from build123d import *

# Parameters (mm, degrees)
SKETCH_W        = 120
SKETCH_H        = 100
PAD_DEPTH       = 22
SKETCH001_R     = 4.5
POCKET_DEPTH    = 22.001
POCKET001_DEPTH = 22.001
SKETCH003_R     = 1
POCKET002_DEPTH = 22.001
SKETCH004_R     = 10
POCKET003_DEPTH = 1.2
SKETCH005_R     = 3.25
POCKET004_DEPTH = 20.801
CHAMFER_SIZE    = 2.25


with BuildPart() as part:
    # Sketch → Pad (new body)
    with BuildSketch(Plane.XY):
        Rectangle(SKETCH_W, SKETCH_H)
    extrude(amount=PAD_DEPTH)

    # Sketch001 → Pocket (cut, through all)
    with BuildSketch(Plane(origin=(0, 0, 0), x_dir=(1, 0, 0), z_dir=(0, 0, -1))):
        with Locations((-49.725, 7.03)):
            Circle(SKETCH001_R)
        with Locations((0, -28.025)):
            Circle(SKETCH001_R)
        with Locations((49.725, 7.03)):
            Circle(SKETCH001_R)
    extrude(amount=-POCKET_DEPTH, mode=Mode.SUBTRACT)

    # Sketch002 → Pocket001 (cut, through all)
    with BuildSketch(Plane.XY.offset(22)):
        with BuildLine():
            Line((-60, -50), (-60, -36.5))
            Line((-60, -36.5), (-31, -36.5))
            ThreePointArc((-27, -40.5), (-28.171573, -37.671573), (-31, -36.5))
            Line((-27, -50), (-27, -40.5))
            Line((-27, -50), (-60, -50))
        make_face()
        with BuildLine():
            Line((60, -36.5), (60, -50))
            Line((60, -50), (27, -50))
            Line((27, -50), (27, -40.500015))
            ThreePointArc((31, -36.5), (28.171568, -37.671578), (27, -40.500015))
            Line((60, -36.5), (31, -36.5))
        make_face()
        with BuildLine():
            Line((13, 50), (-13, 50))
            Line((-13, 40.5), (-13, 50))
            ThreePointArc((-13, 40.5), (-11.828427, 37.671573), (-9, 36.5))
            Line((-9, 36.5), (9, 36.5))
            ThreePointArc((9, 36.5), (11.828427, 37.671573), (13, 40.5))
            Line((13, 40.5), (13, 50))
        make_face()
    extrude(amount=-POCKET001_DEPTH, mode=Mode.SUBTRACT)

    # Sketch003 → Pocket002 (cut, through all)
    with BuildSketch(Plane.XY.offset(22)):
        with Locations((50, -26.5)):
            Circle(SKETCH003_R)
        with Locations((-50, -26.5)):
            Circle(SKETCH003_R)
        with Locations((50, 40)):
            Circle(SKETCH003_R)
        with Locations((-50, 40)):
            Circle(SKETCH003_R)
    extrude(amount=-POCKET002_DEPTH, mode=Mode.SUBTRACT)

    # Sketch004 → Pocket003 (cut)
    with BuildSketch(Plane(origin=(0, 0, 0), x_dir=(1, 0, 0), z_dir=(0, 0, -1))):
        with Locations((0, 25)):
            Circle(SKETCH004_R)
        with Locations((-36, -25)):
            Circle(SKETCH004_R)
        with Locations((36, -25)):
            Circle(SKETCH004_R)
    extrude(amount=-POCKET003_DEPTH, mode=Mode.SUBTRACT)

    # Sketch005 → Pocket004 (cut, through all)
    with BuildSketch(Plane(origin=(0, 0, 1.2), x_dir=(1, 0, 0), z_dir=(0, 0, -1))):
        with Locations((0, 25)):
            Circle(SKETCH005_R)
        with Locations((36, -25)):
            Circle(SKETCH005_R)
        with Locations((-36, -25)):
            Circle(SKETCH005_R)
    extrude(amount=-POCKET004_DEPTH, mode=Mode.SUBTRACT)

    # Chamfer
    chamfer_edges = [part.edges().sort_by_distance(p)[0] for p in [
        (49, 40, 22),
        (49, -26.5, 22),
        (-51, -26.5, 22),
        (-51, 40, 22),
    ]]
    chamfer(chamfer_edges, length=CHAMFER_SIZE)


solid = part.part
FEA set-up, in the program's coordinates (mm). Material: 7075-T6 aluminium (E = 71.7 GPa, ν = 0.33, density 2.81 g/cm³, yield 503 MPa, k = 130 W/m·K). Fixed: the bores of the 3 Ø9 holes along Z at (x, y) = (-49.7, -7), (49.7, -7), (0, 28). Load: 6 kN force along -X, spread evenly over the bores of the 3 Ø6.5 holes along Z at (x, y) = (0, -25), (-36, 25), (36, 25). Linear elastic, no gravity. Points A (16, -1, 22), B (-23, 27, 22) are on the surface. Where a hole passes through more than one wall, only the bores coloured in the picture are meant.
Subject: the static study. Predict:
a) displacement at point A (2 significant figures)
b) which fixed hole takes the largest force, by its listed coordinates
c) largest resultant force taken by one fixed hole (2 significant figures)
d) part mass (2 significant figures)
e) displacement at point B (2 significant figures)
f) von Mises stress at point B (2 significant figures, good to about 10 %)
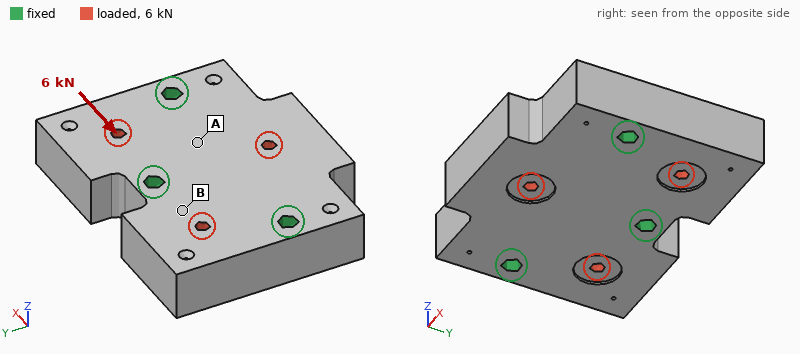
0.78 µm
(0, 28)
2.8 kN
640 g
1.0 µm
3.8 MPa
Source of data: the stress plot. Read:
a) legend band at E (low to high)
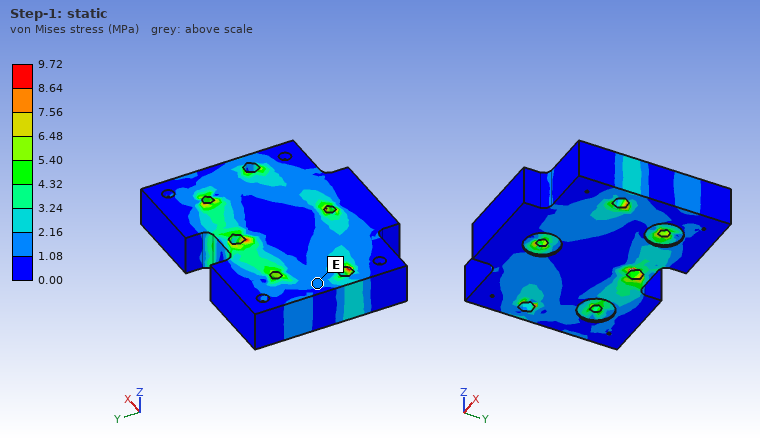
1.08 to 2.16 MPa
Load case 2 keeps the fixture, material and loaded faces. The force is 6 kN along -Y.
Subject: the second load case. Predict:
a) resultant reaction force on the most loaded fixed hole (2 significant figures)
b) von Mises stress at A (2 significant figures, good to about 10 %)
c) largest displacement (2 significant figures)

2.1 kN
1.2 MPa
2.2 µm
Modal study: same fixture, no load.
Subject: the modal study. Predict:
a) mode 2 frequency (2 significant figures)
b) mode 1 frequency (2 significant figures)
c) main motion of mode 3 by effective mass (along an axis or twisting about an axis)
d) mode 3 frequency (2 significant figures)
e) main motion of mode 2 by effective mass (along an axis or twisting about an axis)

7400 Hz
5800 Hz
along Z
7900 Hz
twisting about Y
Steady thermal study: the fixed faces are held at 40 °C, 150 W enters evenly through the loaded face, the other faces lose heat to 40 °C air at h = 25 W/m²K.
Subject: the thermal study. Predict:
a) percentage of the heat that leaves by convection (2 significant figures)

3.4 %
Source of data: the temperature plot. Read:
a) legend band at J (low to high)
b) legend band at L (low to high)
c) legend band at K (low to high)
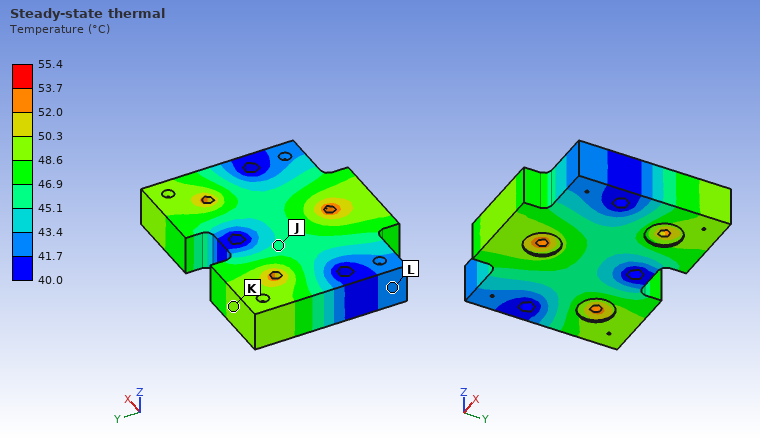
45.1 to 46.9 °C
41.7 to 43.4 °C
48.6 to 50.3 °C
